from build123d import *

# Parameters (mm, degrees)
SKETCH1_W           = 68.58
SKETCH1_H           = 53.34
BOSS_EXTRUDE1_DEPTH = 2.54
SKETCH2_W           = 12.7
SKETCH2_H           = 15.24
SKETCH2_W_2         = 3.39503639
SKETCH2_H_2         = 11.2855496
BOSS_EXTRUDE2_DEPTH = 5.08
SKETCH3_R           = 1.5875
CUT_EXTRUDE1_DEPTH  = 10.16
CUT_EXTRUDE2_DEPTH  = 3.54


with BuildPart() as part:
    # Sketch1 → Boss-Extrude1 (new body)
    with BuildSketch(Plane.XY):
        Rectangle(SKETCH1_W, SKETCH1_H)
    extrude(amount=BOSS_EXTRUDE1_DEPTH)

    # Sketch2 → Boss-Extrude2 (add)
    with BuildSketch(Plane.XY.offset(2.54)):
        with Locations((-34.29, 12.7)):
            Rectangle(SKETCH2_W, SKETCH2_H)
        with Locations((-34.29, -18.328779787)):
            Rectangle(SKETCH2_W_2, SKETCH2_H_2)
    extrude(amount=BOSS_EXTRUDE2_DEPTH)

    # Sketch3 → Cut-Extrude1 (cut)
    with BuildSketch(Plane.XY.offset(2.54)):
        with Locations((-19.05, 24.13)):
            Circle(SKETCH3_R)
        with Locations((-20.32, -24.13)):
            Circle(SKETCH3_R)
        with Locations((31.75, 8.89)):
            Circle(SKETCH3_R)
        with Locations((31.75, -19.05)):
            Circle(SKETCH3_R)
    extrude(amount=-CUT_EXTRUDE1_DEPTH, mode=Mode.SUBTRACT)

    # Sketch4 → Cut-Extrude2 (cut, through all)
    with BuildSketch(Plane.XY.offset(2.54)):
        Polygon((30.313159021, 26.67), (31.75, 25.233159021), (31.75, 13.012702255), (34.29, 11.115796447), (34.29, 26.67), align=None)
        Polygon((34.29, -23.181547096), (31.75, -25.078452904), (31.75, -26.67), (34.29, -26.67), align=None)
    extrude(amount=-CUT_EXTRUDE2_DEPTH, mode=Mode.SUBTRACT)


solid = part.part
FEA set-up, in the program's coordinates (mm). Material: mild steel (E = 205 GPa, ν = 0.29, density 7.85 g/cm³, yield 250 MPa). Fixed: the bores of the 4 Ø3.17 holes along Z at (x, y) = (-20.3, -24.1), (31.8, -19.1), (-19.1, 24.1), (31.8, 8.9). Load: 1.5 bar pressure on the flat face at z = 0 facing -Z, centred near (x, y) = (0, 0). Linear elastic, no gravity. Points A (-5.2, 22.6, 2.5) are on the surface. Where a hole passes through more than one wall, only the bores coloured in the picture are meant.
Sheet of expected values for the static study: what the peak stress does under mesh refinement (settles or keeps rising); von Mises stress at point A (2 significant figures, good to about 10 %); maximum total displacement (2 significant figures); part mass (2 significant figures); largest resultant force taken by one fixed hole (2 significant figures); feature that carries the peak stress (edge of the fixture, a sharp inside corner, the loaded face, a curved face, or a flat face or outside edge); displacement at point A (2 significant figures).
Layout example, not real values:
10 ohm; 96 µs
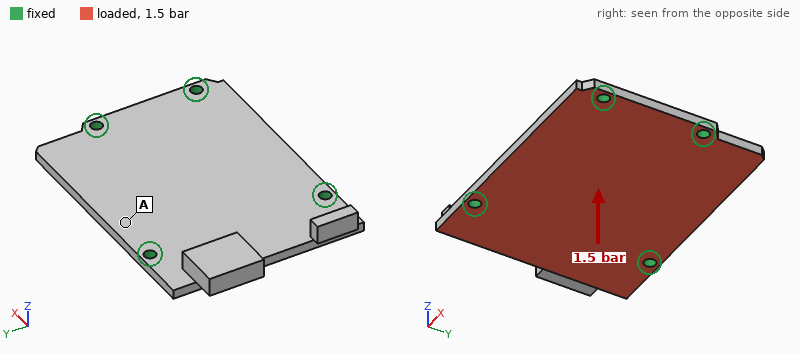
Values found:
keeps rising; 12 MPa; 17 µm; 81 g; 160 N; edge of the fixture; 9.3 µm
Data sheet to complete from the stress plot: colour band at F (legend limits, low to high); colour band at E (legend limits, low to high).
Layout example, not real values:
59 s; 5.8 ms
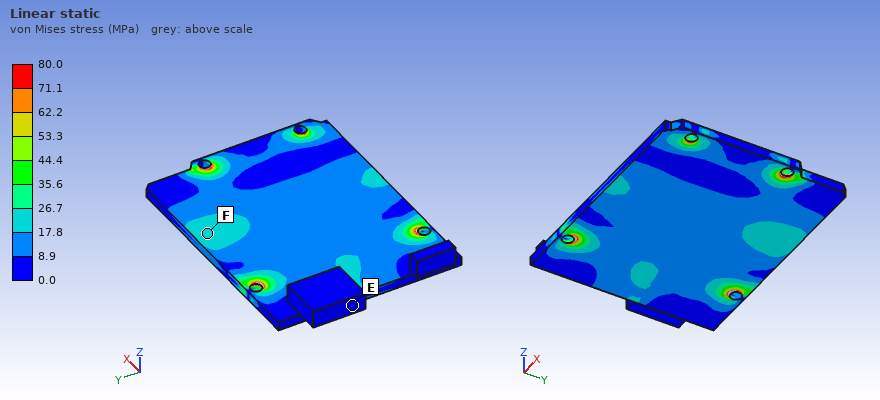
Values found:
17.8 to 26.7 MPa; 0.0 to 8.9 MPa
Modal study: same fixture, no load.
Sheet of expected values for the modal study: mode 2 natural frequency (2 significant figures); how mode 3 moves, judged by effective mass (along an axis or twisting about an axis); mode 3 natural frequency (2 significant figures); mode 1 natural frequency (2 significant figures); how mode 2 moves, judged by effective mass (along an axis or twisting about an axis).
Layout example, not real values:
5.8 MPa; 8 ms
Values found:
3900 Hz; twisting about X; 4900 Hz; 3000 Hz; along Z
